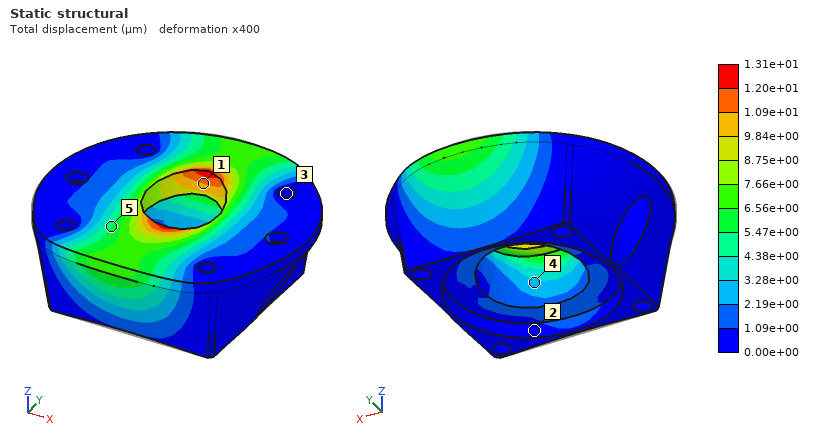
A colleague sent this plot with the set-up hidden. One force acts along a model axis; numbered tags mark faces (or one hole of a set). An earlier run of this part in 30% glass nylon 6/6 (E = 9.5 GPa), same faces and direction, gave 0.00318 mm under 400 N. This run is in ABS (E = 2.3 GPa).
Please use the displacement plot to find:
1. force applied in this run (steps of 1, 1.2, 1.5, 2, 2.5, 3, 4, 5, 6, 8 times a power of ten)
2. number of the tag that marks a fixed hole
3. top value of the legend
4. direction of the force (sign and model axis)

400 N
3
1.31e+01 µm
+Y
